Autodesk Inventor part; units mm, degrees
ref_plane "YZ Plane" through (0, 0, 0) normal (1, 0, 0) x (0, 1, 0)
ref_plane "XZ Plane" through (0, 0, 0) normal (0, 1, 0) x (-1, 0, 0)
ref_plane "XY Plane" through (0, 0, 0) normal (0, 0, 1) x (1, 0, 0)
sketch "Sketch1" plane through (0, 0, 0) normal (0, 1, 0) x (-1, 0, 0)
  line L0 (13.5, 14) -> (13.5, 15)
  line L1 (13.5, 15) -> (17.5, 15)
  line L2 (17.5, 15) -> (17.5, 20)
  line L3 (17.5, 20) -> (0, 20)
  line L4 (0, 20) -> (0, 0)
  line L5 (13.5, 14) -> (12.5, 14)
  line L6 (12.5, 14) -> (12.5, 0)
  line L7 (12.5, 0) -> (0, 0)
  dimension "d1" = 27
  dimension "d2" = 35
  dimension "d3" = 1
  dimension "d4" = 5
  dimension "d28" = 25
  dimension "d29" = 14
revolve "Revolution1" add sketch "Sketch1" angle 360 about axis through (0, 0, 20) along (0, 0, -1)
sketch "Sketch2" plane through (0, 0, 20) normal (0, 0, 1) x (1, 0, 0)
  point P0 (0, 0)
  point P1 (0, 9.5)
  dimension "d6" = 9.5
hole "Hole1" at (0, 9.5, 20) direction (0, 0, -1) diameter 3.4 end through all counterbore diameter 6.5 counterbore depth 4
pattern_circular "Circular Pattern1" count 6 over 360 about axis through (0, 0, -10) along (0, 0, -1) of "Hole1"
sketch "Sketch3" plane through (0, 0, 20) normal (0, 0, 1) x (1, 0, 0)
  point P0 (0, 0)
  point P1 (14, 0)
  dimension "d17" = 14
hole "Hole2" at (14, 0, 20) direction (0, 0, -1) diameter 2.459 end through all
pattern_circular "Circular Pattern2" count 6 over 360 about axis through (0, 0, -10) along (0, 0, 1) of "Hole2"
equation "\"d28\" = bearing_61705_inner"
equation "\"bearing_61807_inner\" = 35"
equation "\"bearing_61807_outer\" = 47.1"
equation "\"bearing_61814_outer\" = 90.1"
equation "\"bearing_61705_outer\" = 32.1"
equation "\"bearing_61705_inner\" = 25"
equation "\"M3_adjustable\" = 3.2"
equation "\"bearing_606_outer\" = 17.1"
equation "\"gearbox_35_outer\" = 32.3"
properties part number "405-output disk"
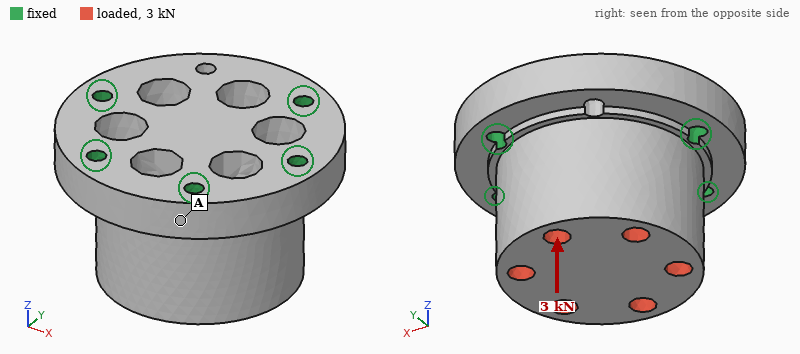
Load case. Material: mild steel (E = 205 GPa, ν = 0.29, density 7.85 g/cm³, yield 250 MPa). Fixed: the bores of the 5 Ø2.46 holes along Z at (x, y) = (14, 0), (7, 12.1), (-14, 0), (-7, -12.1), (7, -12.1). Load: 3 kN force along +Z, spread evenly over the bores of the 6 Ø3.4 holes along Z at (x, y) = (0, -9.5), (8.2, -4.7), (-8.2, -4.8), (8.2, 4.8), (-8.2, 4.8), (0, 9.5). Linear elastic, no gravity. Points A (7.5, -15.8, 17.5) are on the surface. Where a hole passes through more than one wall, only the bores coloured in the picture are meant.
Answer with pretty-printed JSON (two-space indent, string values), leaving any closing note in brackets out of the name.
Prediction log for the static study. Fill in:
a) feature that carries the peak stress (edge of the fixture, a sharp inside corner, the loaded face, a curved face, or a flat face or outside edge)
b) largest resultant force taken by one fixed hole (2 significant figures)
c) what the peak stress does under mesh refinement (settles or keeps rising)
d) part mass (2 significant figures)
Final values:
{
  "feature that carries the peak stress": "edge of the fixture",
  "largest resultant force taken by one fixed hole": "850 N",
  "what the peak stress does under mesh refinement": "keeps rising",
  "part mass": "82 g"
}
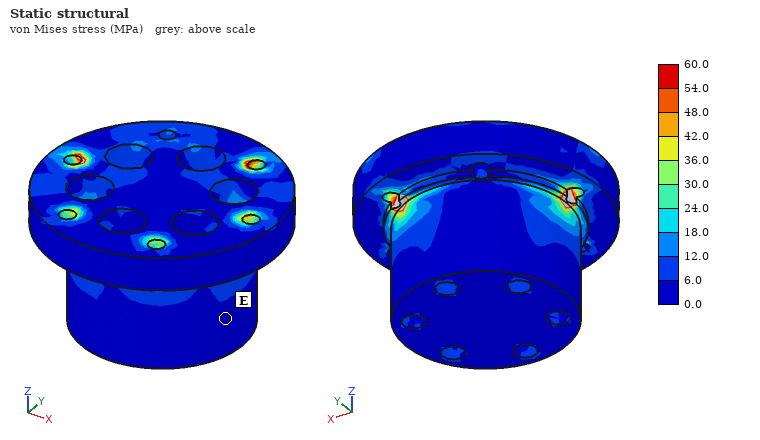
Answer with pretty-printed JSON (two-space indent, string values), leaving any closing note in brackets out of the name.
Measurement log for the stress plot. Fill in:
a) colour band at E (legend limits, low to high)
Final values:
{
  "colour band at E": "0.0 to 6.0 MPa"
}
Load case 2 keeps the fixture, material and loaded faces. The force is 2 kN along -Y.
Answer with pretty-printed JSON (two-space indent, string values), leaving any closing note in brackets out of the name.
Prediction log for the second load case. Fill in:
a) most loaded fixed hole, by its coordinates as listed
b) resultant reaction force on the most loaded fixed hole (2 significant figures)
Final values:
{
  "most loaded fixed hole, by its coordinates as listed": "(7, 12.1)",
  "resultant reaction force on the most loaded fixed hole": "780 N"
}
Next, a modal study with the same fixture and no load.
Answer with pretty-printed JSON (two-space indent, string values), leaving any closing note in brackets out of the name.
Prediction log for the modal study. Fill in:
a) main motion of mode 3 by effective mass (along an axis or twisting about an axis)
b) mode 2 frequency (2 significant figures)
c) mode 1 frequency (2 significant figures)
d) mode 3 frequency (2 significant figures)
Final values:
{
  "main motion of mode 3 by effective mass": "along Z",
  "mode 2 frequency": "29 kHz",
  "mode 1 frequency": "22 kHz",
  "mode 3 frequency": "36 kHz"
}
